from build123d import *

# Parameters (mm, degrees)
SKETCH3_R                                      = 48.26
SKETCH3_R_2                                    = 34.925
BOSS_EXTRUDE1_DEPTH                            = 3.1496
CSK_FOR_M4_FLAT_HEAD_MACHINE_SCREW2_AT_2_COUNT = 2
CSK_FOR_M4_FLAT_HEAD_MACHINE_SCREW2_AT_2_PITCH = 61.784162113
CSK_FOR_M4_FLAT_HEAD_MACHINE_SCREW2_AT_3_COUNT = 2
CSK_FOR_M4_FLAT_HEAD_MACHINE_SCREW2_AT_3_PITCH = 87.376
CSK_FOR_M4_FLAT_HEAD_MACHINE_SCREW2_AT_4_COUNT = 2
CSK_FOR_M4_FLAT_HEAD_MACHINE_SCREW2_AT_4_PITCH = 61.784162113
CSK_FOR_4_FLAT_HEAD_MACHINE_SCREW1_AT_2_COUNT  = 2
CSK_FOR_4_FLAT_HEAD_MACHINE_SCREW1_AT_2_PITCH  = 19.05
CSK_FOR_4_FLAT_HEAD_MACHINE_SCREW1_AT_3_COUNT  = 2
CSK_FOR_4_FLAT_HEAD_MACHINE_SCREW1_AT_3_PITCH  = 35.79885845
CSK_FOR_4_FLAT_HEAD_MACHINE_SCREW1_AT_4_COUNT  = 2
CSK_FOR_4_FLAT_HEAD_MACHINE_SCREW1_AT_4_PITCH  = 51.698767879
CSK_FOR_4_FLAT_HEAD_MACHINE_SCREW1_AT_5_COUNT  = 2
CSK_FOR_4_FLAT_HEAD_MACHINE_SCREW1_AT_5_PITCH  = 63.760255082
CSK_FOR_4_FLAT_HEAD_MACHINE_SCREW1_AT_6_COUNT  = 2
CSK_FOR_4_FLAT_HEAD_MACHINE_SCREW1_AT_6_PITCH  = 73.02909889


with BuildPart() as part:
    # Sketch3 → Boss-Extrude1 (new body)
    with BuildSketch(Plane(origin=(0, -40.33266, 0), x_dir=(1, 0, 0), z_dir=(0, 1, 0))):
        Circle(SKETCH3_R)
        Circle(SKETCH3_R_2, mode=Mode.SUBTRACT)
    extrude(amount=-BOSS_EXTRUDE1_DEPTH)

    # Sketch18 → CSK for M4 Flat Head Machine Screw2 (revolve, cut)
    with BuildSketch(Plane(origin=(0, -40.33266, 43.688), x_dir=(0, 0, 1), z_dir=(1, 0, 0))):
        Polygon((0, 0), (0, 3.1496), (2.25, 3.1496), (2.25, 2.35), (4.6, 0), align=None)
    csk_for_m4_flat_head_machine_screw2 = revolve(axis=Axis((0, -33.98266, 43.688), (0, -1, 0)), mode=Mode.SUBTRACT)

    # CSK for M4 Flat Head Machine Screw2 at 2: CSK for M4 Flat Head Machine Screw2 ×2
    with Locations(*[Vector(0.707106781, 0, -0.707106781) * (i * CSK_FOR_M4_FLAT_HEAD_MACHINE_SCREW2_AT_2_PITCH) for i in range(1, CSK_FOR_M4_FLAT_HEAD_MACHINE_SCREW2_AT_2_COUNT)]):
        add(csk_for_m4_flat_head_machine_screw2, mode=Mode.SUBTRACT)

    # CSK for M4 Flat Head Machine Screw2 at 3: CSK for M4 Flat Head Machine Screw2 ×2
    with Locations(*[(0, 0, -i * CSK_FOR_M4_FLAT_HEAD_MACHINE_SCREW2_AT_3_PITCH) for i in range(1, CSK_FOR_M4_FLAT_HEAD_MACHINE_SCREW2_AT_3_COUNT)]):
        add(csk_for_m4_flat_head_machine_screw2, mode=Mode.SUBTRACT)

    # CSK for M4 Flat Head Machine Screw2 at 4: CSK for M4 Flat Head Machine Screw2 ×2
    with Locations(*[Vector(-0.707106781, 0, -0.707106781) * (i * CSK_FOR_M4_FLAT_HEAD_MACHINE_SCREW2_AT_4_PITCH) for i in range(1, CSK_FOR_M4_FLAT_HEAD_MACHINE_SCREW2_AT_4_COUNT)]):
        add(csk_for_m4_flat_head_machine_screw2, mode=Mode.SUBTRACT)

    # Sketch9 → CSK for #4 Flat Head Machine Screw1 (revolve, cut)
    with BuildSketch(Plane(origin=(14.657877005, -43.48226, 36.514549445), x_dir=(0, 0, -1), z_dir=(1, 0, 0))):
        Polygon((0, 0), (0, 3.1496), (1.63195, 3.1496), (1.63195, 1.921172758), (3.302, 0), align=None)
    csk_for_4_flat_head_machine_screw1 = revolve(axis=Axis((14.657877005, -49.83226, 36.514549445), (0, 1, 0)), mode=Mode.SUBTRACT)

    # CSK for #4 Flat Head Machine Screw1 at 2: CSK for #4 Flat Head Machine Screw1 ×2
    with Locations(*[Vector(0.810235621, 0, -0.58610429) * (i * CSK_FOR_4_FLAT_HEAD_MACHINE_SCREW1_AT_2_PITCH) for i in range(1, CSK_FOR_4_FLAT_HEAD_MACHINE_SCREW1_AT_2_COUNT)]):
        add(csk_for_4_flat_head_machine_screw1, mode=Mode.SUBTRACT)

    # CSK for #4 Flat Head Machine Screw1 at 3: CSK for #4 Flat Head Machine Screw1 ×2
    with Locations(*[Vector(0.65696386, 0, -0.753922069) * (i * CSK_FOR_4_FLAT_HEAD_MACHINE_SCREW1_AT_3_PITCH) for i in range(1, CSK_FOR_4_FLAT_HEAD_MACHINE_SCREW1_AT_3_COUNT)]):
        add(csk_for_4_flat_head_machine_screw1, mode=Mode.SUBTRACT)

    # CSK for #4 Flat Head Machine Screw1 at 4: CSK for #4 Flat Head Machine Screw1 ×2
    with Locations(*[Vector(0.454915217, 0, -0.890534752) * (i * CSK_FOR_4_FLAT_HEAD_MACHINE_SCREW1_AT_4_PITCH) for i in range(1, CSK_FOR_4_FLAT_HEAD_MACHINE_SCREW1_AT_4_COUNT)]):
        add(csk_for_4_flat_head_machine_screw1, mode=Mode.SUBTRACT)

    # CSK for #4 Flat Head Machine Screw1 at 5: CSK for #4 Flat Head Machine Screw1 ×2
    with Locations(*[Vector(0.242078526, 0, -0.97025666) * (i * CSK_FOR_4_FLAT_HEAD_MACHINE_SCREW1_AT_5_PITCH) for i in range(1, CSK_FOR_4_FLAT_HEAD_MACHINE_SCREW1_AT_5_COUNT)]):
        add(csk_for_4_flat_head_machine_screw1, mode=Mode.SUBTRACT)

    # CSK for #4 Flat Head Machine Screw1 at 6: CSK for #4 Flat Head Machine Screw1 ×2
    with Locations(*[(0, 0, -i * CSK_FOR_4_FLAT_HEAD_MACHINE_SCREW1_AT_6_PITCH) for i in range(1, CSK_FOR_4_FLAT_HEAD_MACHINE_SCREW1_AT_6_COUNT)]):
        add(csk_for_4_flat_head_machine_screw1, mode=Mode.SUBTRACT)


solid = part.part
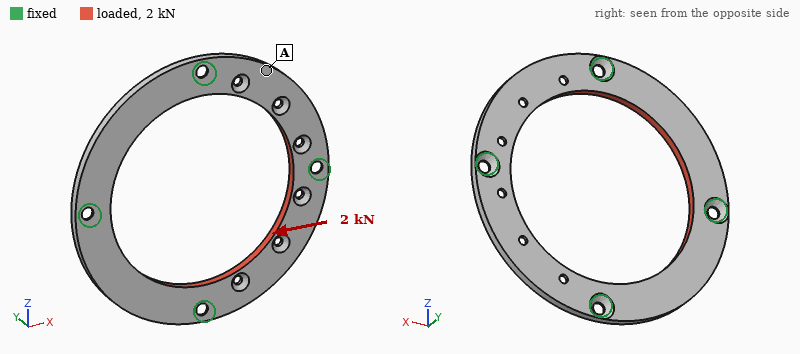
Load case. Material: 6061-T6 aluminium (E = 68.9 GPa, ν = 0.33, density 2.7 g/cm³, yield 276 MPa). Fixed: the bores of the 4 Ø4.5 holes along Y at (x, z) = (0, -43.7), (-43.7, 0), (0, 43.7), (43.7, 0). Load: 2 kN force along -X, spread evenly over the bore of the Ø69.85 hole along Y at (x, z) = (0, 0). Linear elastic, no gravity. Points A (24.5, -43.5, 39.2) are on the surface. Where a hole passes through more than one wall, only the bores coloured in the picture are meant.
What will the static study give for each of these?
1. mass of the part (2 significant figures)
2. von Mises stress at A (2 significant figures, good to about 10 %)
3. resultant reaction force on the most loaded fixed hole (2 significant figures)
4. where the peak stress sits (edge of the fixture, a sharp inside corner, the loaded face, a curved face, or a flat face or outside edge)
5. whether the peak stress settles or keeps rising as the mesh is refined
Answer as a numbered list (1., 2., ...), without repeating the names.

1. 28 g
2. 11 MPa
3. 660 N
4. edge of the fixture
5. keeps rising
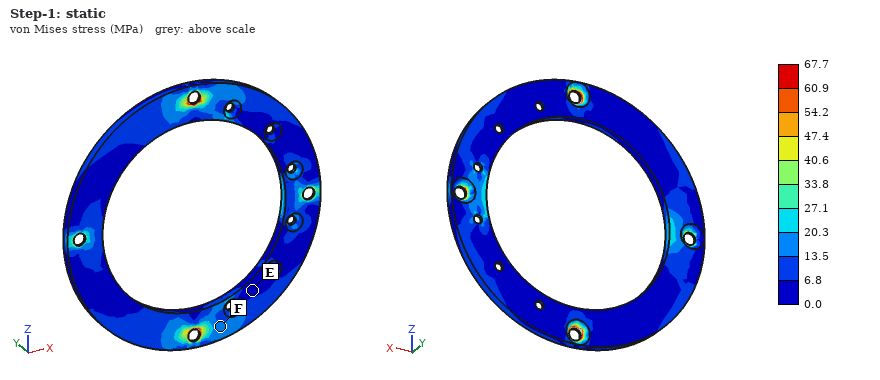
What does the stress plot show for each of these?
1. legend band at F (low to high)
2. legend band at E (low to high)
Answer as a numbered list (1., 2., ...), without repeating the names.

1. 13.5 to 20.3 MPa
2. 0.0 to 6.8 MPa
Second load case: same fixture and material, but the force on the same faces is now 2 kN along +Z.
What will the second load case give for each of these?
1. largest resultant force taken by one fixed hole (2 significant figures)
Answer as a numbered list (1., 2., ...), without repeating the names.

1. 660 N
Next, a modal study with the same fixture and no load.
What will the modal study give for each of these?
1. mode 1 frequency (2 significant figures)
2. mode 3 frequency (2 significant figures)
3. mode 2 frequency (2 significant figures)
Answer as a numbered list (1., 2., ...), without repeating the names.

1. 2500 Hz
2. 2800 Hz
3. 2800 Hz
